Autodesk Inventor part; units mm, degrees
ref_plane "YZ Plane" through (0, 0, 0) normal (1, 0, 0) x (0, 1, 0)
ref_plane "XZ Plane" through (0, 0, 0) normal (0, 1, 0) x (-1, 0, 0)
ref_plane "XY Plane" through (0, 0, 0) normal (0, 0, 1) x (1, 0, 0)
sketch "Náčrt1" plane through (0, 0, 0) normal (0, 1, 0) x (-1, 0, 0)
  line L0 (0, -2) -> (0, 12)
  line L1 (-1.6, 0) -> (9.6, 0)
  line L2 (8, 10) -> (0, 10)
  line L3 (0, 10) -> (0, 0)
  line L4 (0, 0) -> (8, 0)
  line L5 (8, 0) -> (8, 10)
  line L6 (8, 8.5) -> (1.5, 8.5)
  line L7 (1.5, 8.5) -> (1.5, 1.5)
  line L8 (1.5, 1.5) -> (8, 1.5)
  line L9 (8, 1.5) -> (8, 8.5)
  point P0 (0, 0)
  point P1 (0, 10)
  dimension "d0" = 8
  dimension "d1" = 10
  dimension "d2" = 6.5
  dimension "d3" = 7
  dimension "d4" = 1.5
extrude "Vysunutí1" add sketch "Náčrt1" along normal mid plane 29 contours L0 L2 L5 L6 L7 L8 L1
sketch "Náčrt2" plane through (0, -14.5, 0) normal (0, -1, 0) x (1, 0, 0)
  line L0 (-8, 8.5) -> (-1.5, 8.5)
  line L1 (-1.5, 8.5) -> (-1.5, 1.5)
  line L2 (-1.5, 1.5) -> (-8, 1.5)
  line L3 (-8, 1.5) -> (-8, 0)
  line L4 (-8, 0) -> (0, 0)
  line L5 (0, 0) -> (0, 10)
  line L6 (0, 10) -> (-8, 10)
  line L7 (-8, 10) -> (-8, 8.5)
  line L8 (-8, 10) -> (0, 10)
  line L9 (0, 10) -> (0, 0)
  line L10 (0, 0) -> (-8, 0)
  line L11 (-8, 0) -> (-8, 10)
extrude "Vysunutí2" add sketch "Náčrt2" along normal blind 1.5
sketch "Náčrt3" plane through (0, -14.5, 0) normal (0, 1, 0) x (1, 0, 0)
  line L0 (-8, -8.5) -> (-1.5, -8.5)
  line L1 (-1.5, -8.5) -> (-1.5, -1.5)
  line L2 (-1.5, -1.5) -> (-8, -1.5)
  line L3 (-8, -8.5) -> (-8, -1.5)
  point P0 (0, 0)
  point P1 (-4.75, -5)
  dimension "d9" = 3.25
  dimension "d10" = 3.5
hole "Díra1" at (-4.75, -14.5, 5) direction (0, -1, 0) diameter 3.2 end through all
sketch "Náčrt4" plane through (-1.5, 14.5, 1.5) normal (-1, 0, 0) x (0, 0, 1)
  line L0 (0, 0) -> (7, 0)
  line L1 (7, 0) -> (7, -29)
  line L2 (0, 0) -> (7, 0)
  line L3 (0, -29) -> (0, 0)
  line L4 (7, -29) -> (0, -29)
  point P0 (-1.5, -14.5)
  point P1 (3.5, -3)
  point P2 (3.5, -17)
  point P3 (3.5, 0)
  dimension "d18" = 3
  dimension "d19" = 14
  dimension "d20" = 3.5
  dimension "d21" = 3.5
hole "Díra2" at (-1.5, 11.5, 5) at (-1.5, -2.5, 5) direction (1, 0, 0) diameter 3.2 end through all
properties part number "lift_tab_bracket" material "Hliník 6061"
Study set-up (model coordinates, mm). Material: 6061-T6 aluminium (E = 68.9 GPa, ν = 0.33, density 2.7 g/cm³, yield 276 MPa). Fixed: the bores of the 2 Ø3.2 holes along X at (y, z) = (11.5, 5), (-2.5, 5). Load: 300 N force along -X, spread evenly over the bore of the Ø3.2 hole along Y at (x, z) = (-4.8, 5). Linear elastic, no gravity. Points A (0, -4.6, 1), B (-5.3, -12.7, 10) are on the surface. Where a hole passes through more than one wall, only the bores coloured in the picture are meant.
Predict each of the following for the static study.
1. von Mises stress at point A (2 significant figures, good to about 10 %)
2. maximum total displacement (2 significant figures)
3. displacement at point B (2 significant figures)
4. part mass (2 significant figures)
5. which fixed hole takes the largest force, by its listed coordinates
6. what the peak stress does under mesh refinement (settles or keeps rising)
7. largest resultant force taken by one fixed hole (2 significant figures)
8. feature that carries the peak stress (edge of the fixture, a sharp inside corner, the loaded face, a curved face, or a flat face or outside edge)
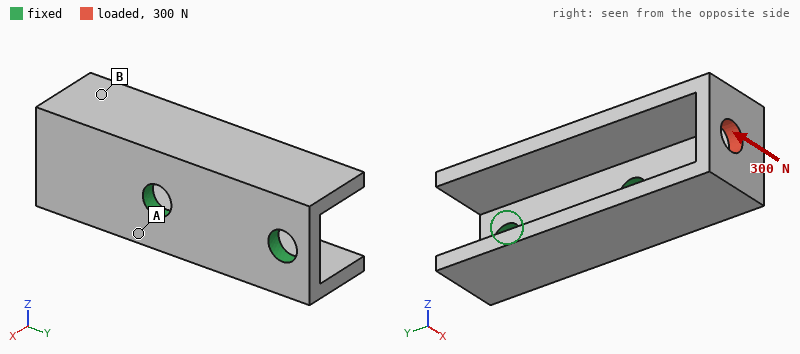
57 MPa
67 µm
49 µm
2.9 g
(-2.5, 5)
keeps rising
560 N
edge of the fixture
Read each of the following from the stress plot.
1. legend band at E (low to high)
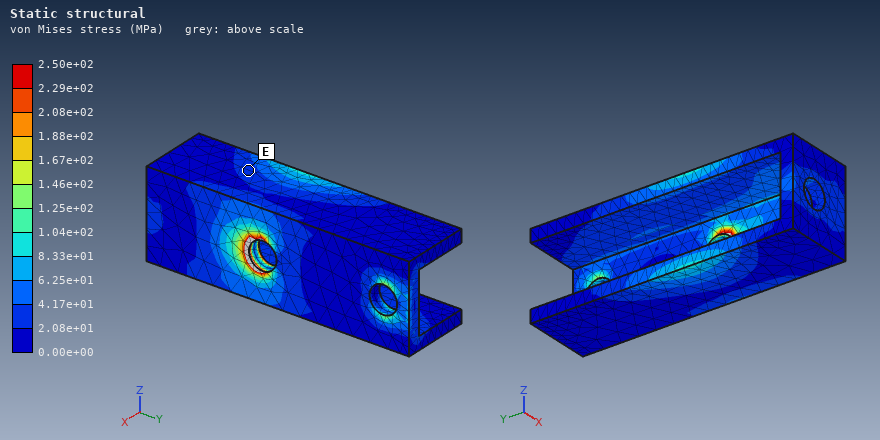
2.08e+01 to 4.17e+01 MPa
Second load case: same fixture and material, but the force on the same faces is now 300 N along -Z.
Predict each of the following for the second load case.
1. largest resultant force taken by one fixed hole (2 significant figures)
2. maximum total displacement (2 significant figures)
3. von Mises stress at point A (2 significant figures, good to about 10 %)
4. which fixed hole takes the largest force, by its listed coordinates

440 N
0.15 mm
89 MPa
(-2.5, 5)
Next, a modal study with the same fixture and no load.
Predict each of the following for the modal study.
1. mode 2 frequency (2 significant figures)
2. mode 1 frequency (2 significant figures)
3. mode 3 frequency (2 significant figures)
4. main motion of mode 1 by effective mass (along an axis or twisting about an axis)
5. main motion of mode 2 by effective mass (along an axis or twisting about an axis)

13 kHz
9600 Hz
15 kHz
along Z
along X
